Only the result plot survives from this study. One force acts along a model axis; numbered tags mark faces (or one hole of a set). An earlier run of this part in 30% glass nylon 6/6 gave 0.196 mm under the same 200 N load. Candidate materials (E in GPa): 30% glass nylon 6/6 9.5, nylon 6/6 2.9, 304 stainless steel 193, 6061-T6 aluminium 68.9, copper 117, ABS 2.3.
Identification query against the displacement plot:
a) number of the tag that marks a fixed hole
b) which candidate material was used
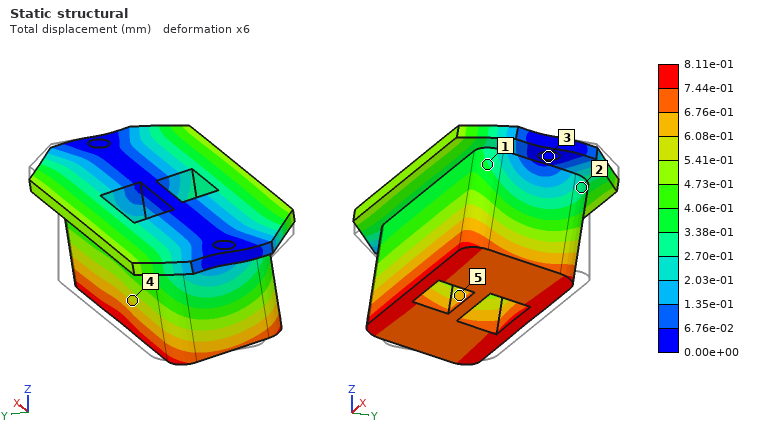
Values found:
3
ABS
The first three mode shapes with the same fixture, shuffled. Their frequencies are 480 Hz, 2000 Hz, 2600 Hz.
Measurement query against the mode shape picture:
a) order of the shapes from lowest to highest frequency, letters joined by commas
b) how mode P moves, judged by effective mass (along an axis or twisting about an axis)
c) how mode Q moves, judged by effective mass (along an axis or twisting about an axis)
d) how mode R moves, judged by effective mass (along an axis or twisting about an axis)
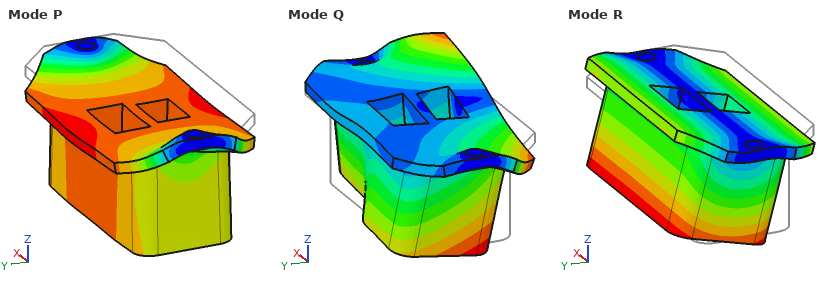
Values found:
R, P, Q
along Z
along X
along Y
